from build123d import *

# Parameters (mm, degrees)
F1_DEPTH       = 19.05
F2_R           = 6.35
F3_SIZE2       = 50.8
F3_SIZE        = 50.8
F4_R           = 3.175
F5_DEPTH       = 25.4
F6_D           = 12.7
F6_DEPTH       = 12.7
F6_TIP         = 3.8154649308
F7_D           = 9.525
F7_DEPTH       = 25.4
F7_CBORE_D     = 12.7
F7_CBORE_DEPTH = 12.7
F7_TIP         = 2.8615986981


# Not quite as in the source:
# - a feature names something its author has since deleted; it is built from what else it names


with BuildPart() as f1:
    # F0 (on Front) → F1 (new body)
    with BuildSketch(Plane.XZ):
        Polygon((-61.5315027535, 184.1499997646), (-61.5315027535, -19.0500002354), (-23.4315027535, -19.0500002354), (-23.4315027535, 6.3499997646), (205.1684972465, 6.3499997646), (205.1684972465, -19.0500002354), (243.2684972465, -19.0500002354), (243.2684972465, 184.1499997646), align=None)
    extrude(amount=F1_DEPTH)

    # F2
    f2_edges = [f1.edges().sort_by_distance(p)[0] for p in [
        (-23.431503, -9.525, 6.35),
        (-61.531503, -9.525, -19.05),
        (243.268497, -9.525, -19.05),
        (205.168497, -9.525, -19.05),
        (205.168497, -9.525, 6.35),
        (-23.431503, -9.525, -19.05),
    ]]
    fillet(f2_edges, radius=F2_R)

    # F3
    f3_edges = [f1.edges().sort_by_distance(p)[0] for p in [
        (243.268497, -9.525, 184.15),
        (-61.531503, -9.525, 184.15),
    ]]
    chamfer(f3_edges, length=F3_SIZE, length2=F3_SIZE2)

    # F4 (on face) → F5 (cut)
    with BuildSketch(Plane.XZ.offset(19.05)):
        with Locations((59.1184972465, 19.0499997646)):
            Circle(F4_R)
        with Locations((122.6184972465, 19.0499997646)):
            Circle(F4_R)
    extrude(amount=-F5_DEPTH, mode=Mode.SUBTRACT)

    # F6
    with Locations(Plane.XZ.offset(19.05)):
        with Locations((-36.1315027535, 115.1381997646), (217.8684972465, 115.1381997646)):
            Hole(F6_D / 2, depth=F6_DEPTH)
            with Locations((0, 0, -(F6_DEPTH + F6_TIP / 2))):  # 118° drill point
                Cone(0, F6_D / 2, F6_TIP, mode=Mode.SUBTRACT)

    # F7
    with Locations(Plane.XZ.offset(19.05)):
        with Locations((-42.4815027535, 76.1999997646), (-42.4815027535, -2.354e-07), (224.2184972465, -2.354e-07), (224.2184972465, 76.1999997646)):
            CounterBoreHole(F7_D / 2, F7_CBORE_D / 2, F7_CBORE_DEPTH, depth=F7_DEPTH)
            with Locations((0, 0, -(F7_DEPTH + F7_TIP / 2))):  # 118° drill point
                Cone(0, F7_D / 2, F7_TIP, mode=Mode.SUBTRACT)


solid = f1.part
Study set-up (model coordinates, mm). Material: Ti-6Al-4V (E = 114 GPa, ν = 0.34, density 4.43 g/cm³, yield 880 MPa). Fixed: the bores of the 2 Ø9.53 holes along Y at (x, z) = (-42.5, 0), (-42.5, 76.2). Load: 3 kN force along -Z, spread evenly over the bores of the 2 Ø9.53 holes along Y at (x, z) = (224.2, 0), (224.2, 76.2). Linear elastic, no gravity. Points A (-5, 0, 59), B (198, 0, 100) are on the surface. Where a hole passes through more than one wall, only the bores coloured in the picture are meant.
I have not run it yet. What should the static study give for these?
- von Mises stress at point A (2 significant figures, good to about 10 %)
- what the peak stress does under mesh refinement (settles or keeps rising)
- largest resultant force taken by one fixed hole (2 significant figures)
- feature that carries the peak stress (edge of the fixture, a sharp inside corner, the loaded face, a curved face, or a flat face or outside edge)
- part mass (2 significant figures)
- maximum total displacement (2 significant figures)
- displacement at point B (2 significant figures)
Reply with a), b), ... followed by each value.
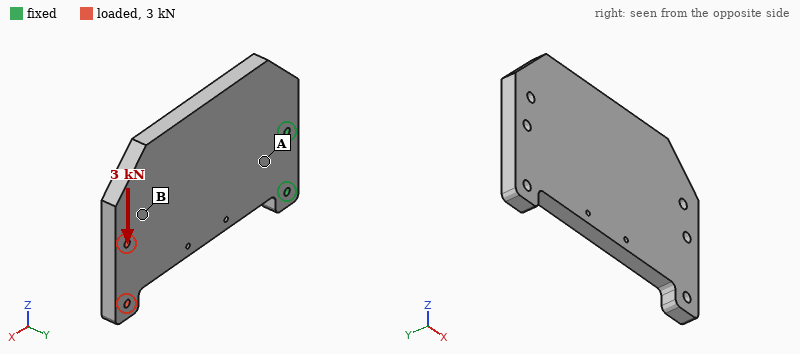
a) 14 MPa
b) keeps rising
c) 10 kN
d) edge of the fixture
e) 4.5 kg
f) 0.18 mm
g) 0.14 mm
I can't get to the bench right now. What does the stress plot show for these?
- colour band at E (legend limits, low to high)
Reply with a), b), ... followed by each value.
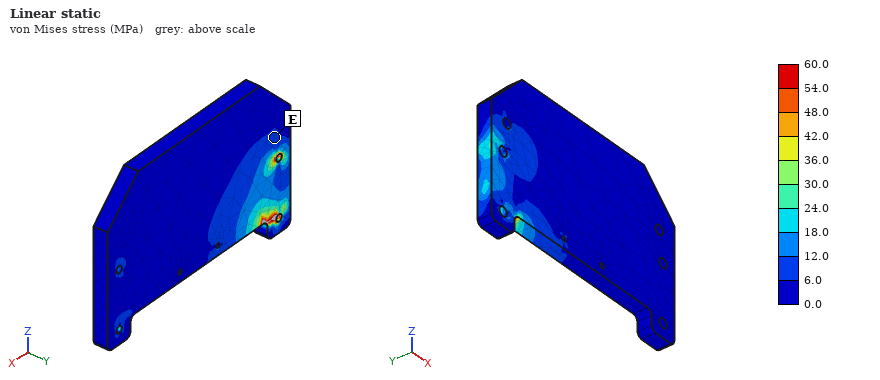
a) 6.0 to 12.0 MPa
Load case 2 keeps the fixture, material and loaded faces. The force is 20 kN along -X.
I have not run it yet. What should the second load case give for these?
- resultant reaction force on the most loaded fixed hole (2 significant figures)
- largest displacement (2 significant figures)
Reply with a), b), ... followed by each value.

a) 10 kN
b) 0.55 mm
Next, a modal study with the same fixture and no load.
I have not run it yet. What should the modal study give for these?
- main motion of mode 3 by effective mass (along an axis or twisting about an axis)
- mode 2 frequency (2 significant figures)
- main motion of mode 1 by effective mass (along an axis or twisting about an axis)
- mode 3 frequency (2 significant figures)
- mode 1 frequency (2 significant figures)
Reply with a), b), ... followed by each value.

a) along Z
b) 460 Hz
c) along Y
d) 610 Hz
e) 110 Hz
